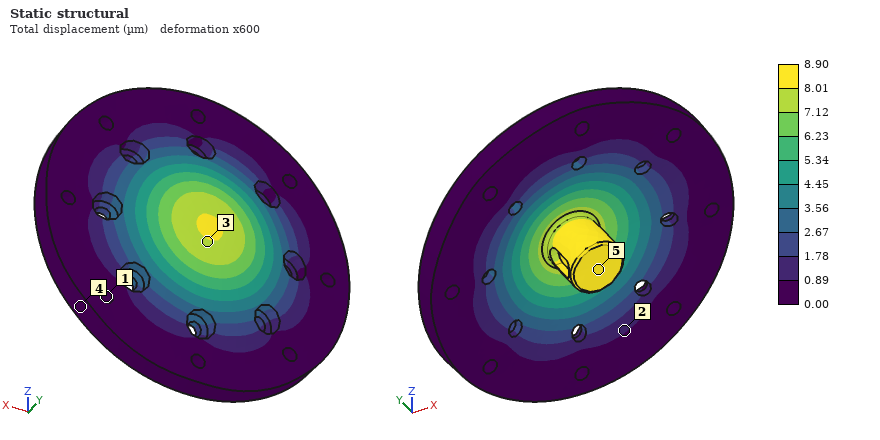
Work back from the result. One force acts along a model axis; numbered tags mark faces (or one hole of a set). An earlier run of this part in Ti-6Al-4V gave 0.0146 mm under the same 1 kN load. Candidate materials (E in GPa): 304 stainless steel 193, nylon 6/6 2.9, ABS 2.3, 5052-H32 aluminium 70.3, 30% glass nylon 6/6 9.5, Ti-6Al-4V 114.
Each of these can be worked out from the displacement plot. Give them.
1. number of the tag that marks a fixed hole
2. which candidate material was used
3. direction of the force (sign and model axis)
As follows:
1
304 stainless steel
+Y
